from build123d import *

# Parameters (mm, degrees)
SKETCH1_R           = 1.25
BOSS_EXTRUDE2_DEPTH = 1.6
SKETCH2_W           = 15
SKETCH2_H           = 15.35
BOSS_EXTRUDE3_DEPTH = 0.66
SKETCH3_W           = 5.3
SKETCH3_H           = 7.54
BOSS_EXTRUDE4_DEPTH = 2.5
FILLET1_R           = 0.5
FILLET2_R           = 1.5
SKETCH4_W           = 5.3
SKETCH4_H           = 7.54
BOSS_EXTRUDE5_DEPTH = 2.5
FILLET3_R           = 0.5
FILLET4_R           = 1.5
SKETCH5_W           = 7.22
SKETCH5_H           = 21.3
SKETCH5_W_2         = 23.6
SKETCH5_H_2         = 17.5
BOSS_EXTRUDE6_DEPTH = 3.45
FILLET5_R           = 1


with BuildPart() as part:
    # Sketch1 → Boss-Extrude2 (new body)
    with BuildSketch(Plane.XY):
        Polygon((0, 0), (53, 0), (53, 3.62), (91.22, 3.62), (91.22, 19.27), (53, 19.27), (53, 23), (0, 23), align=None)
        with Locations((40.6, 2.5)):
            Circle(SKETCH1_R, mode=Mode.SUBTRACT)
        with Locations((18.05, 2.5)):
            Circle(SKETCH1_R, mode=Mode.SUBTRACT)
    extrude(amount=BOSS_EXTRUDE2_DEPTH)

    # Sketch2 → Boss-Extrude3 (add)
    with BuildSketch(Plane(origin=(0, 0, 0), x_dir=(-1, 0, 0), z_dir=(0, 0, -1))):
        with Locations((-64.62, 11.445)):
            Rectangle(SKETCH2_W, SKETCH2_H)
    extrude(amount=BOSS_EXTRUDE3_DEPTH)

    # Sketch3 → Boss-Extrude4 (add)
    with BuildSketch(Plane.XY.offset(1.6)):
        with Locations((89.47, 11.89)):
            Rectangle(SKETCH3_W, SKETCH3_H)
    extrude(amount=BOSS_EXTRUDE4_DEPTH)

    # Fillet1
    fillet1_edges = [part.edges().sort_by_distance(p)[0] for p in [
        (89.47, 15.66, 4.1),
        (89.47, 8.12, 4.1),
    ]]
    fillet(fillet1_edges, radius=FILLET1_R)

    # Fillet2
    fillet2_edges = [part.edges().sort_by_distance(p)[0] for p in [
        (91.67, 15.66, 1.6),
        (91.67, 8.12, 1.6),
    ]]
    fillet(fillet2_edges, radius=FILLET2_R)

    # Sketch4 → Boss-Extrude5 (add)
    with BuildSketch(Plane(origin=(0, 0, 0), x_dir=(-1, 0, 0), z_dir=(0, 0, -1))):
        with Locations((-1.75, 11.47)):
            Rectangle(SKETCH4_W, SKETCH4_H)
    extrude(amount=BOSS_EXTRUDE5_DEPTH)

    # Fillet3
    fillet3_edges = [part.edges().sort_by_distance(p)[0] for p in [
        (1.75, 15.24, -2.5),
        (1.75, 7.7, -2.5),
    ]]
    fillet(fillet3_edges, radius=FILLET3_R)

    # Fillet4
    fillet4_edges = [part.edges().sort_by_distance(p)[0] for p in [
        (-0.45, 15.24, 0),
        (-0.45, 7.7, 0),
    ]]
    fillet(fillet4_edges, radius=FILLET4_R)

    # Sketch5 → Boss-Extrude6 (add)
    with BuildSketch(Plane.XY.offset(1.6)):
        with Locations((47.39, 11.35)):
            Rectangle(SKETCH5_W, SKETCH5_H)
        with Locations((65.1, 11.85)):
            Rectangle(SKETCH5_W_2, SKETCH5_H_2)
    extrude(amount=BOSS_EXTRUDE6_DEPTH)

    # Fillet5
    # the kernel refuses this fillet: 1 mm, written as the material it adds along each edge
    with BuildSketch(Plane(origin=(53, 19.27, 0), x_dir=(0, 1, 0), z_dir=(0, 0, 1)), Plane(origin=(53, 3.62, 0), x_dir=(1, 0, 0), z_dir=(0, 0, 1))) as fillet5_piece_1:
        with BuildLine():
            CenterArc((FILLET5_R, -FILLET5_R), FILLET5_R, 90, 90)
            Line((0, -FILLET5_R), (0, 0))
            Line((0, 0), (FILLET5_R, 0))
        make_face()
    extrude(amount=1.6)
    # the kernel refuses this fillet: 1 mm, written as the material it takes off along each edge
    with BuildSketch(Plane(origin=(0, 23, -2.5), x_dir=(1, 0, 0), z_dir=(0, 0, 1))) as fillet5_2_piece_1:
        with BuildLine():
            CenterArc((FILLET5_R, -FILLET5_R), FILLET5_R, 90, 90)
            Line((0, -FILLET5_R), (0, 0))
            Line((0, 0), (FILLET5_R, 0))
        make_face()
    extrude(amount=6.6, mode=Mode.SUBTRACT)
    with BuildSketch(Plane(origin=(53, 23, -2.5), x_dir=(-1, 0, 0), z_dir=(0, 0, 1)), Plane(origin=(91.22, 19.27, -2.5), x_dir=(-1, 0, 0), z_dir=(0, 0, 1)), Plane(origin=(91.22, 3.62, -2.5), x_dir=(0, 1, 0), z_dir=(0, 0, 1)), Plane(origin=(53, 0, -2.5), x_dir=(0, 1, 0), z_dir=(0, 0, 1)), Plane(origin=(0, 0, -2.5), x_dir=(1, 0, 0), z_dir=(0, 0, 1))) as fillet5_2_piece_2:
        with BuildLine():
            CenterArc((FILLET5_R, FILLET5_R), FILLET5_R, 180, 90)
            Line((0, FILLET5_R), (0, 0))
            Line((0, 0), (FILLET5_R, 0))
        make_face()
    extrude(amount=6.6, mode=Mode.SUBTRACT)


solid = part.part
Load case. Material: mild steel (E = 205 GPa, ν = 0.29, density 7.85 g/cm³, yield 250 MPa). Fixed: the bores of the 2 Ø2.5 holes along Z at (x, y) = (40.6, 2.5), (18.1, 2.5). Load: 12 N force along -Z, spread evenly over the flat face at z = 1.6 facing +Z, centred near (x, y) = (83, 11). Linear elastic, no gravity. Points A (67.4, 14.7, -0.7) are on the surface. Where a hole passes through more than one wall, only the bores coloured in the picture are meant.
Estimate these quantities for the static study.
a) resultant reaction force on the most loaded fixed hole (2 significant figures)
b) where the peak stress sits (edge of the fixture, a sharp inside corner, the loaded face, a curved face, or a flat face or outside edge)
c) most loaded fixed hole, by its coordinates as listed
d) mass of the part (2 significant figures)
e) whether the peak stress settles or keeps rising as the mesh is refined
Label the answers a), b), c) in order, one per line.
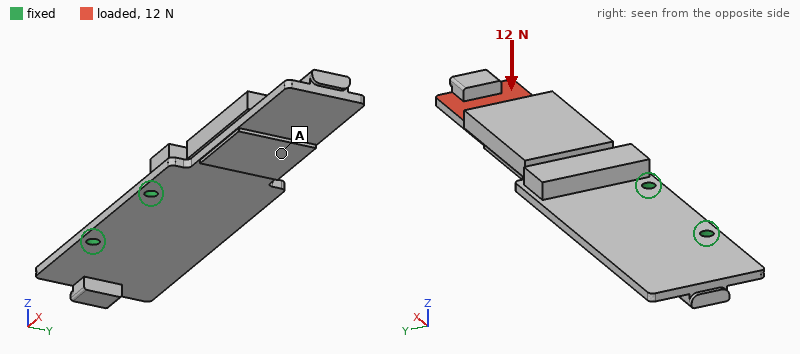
a) 21 N
b) edge of the fixture
c) (40.6, 2.5)
d) 41 g
e) keeps rising
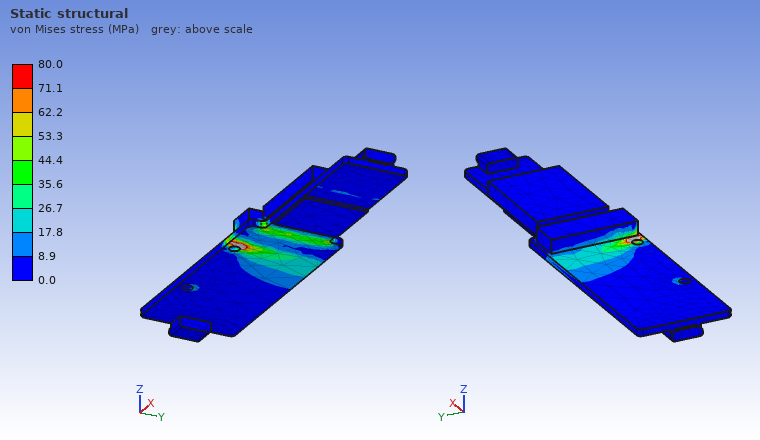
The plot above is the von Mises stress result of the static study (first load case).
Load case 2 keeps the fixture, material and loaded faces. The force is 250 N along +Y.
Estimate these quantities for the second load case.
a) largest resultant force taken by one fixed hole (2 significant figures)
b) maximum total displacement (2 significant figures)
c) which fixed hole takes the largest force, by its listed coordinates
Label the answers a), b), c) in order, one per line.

a) 740 N
b) 58 µm
c) (40.6, 2.5)
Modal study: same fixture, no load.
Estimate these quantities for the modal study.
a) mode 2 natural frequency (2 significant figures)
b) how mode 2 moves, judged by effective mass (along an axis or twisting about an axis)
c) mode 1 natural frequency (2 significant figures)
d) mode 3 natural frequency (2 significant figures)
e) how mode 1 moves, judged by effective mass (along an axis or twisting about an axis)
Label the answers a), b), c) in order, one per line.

a) 2200 Hz
b) along Z
c) 520 Hz
d) 2400 Hz
e) along Z
